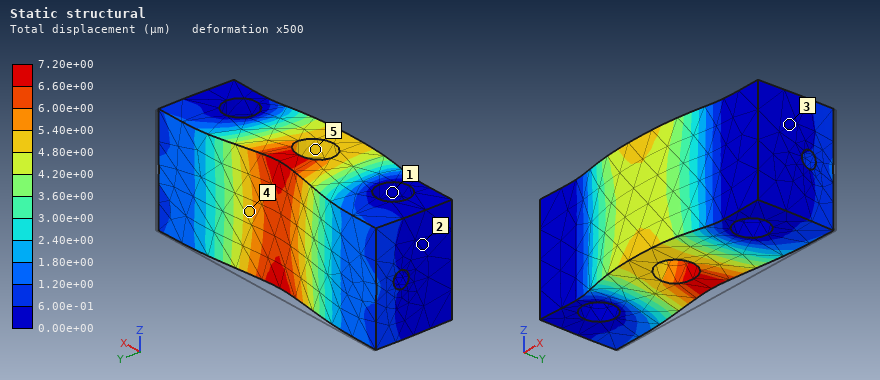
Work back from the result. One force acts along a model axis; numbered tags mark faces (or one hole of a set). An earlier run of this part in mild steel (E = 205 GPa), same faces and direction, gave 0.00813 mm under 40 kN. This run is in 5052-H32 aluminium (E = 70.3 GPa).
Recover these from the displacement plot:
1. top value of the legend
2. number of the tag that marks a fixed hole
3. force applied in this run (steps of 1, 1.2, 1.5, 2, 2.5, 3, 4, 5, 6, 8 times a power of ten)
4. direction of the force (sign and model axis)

7.20e+00 µm
1
12 kN
-Y
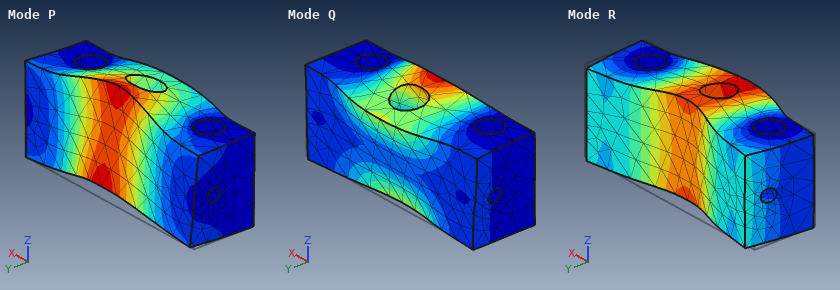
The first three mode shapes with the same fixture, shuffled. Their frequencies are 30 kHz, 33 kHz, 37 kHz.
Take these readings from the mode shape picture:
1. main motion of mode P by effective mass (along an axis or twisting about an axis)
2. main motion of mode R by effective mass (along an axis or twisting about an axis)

along Z
along Y
